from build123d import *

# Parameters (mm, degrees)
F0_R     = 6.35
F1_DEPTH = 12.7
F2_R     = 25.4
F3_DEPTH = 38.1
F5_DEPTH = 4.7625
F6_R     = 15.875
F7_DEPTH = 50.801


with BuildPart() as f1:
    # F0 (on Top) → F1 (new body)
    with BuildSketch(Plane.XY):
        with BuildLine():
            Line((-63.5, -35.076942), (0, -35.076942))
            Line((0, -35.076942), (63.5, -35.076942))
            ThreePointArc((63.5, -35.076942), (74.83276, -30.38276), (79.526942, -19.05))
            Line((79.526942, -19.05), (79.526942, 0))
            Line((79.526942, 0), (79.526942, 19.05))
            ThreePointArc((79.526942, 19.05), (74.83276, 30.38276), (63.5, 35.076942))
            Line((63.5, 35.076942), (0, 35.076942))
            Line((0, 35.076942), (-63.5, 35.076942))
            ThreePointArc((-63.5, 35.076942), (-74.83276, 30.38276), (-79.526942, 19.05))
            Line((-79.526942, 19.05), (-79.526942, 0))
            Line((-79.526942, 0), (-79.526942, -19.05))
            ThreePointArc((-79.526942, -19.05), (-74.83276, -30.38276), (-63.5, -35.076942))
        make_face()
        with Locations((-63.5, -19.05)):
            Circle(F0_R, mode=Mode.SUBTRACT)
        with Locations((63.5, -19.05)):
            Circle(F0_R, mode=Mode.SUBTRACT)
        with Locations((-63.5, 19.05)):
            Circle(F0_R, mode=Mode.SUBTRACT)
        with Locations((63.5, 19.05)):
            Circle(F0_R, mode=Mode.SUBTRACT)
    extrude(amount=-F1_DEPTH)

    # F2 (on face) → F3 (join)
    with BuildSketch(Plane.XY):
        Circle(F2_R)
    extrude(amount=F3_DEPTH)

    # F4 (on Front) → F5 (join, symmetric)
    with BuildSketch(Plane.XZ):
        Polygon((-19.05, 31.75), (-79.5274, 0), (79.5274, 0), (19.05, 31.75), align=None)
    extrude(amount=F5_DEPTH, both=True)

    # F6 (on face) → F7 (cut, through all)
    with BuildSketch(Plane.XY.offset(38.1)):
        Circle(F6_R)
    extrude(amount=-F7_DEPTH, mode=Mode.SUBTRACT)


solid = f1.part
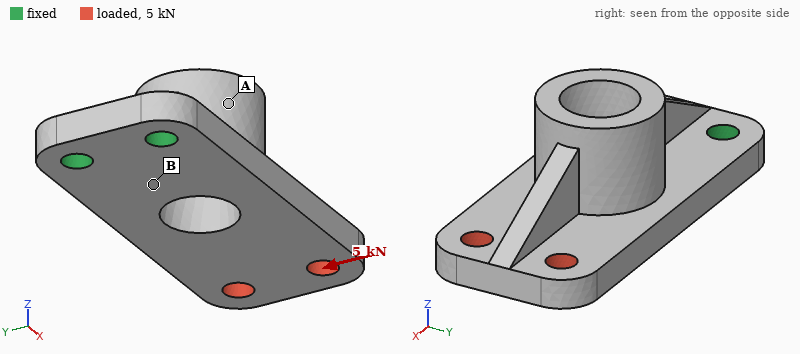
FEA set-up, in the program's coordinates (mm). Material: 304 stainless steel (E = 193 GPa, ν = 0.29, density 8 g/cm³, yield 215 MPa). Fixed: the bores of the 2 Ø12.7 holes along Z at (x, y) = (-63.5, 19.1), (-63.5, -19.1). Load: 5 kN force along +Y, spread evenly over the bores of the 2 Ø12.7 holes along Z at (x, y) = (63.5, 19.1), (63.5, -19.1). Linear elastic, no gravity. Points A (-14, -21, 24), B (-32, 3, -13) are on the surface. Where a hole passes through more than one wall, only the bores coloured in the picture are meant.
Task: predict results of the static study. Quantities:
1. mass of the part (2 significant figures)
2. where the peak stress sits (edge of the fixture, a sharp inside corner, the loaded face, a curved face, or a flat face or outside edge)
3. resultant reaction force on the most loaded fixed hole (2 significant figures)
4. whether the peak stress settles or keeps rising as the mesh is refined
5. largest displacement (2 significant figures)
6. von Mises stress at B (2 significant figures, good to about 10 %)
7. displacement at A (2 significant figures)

1.5 kg
edge of the fixture
14 kN
keeps rising
80 µm
28 MPa
17 µm
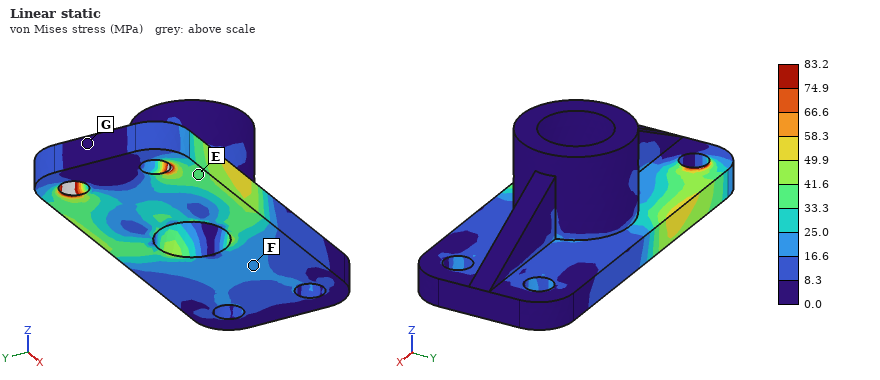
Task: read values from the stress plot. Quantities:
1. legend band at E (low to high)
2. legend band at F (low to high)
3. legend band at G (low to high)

33.3 to 41.6 MPa
16.6 to 25.0 MPa
0.0 to 8.3 MPa
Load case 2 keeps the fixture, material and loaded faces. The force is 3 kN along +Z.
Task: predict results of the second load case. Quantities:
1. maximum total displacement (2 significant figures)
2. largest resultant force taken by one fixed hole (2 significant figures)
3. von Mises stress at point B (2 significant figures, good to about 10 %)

0.37 mm
1.5 kN
50 MPa
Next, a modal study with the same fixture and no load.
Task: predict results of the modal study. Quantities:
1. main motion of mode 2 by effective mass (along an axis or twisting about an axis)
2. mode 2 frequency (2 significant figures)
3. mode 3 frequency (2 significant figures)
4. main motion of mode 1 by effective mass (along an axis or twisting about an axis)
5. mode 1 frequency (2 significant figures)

along Y
2000 Hz
2300 Hz
along Z
730 Hz
